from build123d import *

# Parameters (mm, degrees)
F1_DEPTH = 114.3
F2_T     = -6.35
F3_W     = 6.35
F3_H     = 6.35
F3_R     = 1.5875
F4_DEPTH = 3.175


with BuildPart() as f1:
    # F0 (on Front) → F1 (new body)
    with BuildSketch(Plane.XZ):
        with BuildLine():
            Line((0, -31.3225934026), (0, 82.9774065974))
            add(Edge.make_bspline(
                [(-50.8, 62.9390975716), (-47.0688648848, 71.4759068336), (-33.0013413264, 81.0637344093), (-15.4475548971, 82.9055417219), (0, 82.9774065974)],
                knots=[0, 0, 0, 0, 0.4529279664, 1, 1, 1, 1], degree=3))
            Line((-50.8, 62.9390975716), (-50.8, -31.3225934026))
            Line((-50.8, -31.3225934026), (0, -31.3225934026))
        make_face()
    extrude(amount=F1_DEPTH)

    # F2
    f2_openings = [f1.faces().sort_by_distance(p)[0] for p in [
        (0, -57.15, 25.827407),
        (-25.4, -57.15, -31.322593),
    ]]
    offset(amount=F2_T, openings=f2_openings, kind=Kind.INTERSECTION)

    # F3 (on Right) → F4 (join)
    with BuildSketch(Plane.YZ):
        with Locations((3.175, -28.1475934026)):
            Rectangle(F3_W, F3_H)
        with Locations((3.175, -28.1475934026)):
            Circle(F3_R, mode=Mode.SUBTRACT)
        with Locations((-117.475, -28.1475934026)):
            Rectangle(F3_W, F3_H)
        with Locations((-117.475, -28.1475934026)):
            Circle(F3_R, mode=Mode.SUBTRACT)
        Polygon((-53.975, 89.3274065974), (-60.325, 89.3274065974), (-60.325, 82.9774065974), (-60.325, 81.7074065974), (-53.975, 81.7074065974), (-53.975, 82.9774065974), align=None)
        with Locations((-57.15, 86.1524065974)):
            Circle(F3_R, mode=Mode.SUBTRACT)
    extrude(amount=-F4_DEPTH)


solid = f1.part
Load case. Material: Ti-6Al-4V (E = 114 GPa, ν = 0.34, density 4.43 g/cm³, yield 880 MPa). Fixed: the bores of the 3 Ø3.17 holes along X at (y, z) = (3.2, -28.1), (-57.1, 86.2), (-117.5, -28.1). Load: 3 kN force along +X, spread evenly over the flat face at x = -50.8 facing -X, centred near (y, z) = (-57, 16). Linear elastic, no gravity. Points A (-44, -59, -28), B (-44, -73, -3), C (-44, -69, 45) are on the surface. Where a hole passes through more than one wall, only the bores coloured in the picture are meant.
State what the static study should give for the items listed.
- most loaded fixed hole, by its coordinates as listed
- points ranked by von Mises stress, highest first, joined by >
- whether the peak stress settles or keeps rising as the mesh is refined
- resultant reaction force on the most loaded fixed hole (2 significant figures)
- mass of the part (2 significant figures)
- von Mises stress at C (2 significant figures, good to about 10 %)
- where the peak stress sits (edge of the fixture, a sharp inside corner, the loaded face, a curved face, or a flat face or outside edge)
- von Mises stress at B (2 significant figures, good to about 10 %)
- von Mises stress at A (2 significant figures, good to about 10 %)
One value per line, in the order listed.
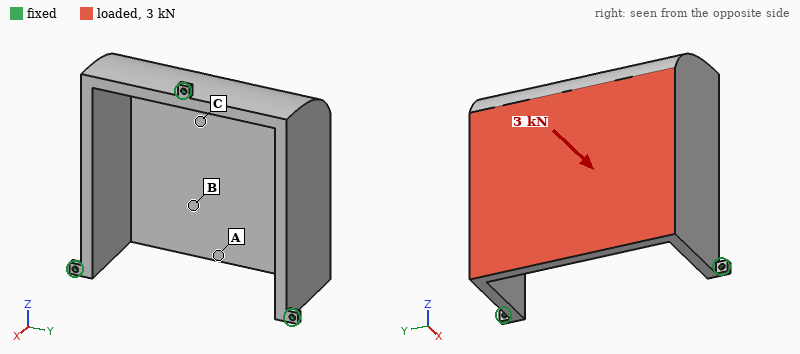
(-57.1, 86.2)
A > B > C
keeps rising
1.3 kN
740 g
7.9 MPa
edge of the fixture
17 MPa
26 MPa
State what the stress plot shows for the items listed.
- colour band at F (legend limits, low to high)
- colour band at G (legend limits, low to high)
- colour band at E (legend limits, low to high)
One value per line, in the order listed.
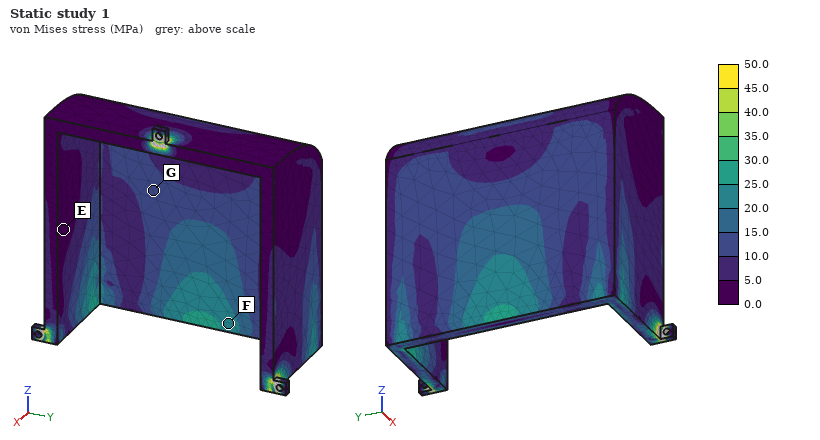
20.0 to 25.0 MPa
10.0 to 15.0 MPa
0.0 to 5.0 MPa
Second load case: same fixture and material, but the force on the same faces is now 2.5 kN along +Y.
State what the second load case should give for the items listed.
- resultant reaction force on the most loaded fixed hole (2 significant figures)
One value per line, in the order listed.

1.4 kN
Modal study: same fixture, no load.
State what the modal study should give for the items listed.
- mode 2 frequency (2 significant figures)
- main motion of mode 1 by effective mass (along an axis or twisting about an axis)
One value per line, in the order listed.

2100 Hz
along Y
